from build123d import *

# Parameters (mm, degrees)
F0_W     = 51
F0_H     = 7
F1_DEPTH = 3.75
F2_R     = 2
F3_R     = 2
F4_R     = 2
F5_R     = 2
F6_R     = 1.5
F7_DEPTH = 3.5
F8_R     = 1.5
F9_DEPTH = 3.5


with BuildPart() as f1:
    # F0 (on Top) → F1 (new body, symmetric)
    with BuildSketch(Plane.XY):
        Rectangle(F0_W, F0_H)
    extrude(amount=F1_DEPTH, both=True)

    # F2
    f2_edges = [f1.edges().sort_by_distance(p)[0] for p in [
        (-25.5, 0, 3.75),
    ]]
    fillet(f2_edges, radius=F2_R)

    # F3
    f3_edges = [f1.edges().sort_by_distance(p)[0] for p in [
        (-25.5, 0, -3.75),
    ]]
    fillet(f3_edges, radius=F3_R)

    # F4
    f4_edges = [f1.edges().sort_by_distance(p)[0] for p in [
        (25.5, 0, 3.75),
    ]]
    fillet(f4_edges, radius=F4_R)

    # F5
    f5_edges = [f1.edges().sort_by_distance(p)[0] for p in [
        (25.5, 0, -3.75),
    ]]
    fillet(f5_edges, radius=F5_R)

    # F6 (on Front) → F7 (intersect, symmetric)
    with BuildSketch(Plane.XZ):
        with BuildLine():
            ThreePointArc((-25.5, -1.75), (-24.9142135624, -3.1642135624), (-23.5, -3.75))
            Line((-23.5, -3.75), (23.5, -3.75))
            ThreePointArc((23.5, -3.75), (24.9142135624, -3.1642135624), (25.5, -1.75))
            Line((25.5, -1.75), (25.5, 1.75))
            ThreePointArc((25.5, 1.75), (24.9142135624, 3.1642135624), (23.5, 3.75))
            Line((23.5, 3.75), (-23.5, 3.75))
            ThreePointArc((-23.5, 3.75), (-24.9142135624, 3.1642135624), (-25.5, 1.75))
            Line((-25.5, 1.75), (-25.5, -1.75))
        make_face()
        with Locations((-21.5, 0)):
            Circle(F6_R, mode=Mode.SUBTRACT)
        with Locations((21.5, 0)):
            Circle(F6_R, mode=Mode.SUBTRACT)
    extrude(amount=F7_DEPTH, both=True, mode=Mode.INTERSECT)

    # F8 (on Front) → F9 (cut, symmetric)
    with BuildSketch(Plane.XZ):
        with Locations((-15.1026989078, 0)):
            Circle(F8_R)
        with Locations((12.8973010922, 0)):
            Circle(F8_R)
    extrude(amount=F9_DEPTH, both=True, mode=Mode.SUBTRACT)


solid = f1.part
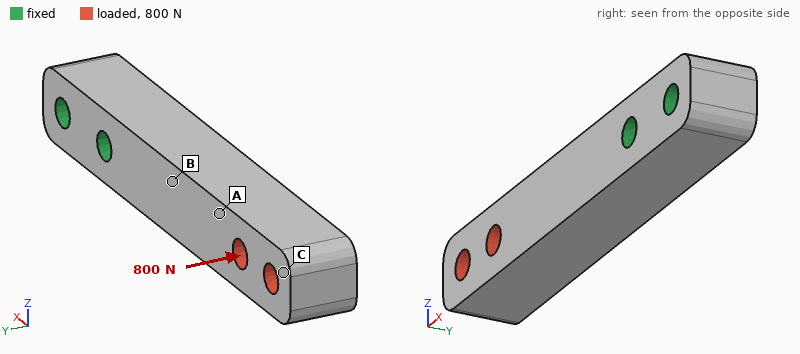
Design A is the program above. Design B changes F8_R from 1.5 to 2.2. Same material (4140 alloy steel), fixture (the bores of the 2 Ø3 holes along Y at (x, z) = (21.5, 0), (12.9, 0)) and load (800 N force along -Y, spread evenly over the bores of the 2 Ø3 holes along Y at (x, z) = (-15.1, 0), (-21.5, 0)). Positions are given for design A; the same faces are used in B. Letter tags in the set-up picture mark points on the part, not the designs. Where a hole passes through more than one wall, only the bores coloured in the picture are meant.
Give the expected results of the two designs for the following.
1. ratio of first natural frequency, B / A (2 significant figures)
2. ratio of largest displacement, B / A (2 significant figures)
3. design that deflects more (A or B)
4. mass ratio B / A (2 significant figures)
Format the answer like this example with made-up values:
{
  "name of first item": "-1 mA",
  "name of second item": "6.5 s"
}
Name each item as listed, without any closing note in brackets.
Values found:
{
  "ratio of first natural frequency, B / A": "1.1",
  "ratio of largest displacement, B / A": "0.90",
  "design that deflects more": "A",
  "mass ratio B / A": "0.95"
}
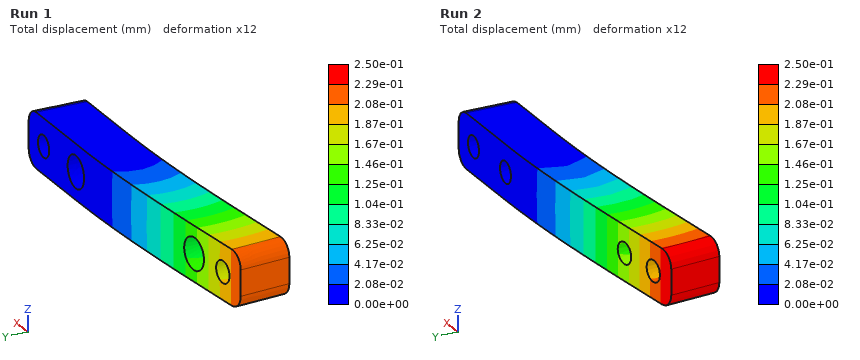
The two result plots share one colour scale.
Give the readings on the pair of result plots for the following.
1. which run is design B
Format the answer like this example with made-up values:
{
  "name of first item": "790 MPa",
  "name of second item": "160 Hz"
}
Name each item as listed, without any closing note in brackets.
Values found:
{
  "which run is design B": "Run 1"
}
